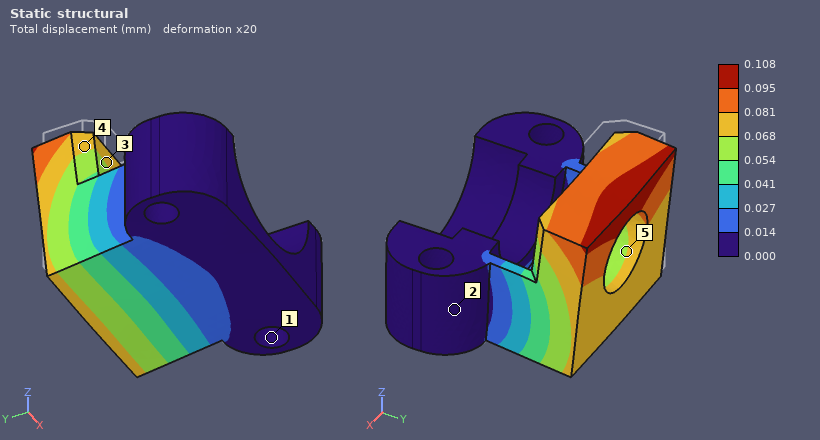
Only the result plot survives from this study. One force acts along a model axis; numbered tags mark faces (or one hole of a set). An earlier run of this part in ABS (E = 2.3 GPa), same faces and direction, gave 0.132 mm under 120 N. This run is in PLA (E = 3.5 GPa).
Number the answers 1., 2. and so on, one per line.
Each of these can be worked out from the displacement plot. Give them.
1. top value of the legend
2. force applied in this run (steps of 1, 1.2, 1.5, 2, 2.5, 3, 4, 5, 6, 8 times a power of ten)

1. 0.108 mm
2. 150 N
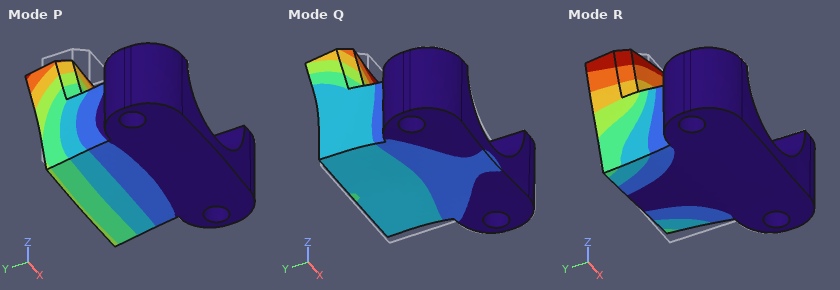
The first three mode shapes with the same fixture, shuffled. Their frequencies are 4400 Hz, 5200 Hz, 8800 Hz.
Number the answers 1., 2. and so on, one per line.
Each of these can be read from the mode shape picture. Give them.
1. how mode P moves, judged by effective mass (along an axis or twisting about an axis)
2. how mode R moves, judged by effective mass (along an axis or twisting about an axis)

1. along Z
2. along X
